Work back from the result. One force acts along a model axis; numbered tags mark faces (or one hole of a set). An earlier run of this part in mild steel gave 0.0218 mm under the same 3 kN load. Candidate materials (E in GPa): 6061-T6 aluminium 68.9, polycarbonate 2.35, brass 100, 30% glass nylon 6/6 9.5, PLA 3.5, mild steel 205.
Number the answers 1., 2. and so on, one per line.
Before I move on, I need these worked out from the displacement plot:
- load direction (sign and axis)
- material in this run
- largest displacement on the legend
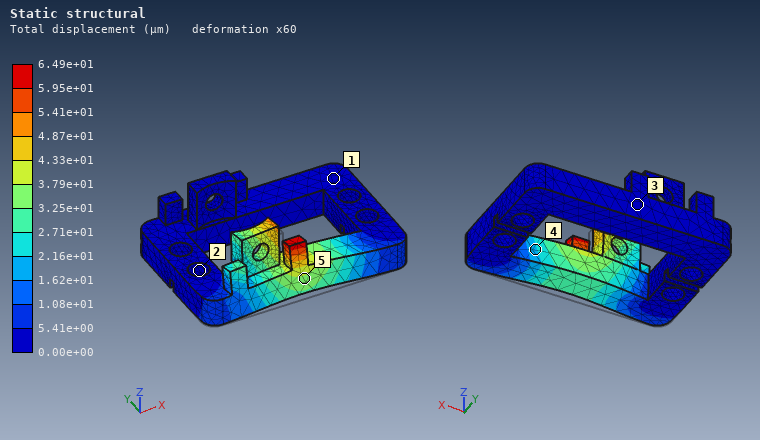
1. +Y
2. 6061-T6 aluminium
3. 6.49e+01 µm
